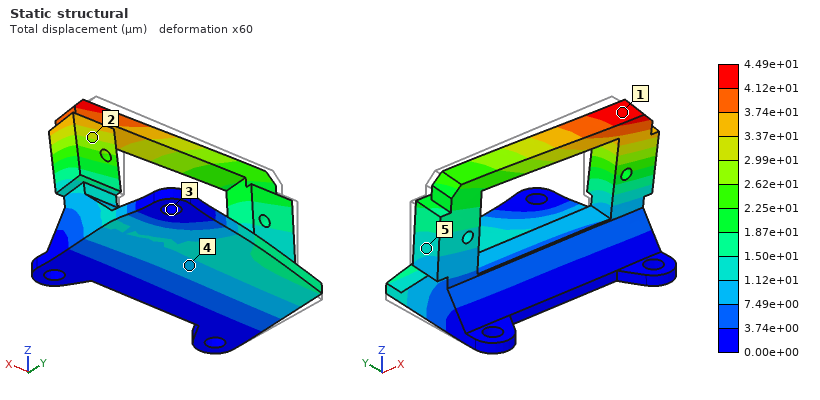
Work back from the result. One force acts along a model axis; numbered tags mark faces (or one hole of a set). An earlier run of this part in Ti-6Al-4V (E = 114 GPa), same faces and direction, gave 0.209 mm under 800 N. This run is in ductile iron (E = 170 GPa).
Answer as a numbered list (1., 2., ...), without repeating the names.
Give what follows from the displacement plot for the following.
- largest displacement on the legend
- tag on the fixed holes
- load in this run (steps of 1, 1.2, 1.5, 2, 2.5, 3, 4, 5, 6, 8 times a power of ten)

1. 4.49e+01 µm
2. 3
3. 250 N
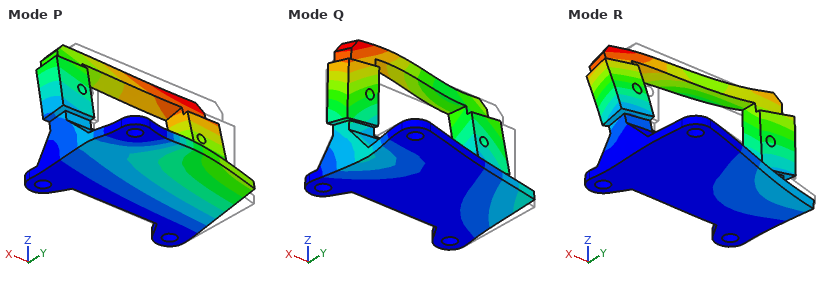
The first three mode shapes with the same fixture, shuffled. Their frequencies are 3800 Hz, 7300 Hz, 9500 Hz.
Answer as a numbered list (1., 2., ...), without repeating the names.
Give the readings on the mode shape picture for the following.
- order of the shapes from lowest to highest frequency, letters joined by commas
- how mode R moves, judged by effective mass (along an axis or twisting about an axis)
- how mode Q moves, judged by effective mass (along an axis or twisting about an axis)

1. P, Q, R
2. along X
3. along X
